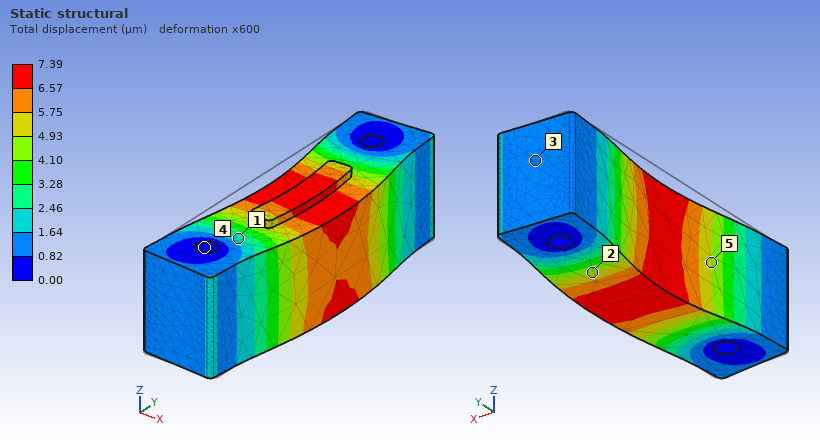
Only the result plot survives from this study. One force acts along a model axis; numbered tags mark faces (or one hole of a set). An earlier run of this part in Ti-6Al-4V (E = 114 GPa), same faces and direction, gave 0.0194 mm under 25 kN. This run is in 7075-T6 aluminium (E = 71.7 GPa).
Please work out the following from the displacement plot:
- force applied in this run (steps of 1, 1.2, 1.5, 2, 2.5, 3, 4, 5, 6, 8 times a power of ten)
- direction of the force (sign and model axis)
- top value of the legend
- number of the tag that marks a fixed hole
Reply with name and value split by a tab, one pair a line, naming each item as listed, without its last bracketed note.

force applied in this run	6 kN
direction of the force	+X
top value of the legend	7.39 µm
number of the tag that marks a fixed hole	4
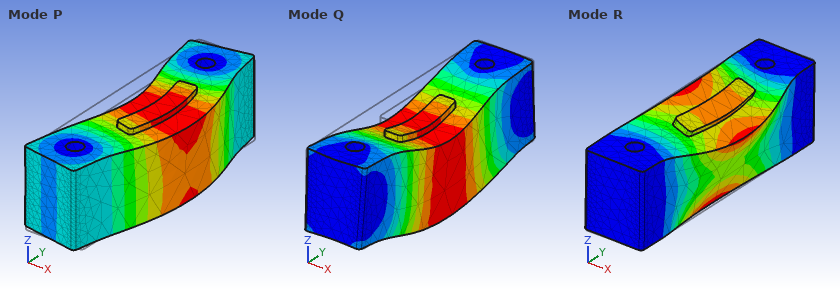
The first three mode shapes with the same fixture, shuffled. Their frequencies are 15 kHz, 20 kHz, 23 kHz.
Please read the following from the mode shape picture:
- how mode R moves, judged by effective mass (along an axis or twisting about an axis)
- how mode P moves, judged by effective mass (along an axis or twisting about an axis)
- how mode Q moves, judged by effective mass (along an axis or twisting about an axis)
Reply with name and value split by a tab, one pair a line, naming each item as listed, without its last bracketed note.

how mode R moves, judged by effective mass	twisting about Y
how mode P moves, judged by effective mass	along X
how mode Q moves, judged by effective mass	along Z
